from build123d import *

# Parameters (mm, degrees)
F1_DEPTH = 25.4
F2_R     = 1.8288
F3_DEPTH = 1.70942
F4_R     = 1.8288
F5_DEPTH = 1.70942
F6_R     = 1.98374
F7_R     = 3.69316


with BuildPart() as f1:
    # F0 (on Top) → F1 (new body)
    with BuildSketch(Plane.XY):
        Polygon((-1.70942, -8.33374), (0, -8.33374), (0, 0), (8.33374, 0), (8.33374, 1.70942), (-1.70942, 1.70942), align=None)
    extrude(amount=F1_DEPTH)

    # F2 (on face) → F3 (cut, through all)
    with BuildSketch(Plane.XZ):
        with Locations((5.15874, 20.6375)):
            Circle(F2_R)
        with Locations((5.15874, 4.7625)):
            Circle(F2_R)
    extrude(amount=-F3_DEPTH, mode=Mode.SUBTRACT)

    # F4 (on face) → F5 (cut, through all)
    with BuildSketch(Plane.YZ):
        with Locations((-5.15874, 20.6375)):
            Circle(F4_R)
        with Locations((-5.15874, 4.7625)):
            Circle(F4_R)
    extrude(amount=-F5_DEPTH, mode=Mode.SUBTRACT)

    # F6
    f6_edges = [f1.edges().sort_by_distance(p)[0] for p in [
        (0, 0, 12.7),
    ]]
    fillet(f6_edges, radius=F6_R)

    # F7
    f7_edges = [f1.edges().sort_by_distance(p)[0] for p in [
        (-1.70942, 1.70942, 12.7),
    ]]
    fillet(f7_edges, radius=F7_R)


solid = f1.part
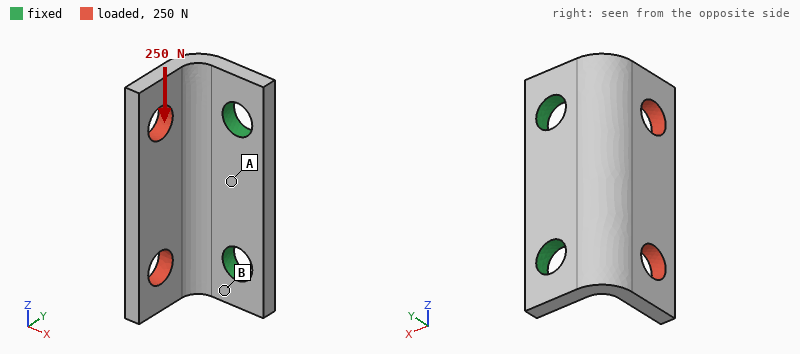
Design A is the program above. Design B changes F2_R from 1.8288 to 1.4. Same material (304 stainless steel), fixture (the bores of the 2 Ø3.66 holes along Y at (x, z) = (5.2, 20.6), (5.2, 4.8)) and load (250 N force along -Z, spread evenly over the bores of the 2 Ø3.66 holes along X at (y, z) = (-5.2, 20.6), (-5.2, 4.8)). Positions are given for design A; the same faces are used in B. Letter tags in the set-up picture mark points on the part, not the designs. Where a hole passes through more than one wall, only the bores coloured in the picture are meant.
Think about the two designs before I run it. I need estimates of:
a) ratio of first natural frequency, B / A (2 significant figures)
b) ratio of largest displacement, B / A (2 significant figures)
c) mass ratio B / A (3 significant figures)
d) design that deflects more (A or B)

0.93
1.2
1.02
B
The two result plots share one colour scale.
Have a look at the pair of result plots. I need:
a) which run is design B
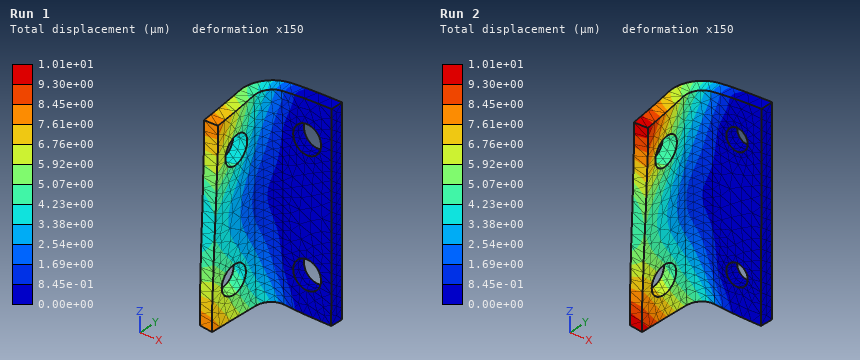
Run 2
